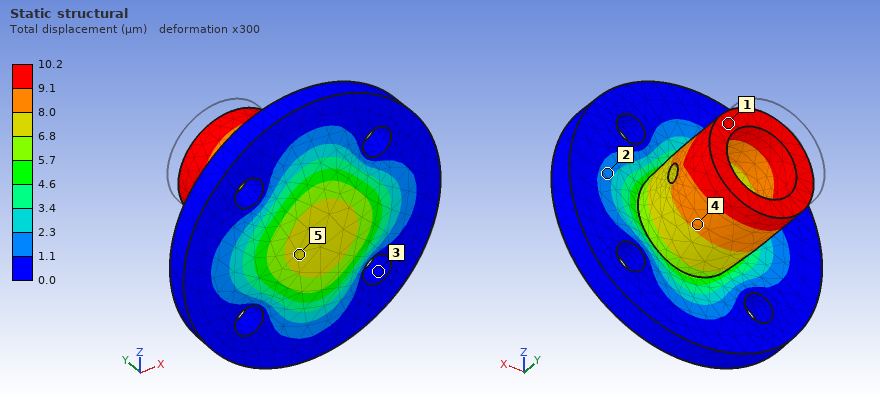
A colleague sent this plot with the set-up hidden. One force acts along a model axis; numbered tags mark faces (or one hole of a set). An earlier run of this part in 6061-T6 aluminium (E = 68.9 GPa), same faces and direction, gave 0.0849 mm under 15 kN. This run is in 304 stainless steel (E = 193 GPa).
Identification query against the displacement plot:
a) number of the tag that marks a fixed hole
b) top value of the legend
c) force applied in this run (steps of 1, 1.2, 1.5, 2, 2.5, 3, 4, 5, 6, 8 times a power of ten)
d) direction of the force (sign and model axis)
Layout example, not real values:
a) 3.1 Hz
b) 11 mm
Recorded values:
a) 3
b) 10.2 µm
c) 5 kN
d) -Y
